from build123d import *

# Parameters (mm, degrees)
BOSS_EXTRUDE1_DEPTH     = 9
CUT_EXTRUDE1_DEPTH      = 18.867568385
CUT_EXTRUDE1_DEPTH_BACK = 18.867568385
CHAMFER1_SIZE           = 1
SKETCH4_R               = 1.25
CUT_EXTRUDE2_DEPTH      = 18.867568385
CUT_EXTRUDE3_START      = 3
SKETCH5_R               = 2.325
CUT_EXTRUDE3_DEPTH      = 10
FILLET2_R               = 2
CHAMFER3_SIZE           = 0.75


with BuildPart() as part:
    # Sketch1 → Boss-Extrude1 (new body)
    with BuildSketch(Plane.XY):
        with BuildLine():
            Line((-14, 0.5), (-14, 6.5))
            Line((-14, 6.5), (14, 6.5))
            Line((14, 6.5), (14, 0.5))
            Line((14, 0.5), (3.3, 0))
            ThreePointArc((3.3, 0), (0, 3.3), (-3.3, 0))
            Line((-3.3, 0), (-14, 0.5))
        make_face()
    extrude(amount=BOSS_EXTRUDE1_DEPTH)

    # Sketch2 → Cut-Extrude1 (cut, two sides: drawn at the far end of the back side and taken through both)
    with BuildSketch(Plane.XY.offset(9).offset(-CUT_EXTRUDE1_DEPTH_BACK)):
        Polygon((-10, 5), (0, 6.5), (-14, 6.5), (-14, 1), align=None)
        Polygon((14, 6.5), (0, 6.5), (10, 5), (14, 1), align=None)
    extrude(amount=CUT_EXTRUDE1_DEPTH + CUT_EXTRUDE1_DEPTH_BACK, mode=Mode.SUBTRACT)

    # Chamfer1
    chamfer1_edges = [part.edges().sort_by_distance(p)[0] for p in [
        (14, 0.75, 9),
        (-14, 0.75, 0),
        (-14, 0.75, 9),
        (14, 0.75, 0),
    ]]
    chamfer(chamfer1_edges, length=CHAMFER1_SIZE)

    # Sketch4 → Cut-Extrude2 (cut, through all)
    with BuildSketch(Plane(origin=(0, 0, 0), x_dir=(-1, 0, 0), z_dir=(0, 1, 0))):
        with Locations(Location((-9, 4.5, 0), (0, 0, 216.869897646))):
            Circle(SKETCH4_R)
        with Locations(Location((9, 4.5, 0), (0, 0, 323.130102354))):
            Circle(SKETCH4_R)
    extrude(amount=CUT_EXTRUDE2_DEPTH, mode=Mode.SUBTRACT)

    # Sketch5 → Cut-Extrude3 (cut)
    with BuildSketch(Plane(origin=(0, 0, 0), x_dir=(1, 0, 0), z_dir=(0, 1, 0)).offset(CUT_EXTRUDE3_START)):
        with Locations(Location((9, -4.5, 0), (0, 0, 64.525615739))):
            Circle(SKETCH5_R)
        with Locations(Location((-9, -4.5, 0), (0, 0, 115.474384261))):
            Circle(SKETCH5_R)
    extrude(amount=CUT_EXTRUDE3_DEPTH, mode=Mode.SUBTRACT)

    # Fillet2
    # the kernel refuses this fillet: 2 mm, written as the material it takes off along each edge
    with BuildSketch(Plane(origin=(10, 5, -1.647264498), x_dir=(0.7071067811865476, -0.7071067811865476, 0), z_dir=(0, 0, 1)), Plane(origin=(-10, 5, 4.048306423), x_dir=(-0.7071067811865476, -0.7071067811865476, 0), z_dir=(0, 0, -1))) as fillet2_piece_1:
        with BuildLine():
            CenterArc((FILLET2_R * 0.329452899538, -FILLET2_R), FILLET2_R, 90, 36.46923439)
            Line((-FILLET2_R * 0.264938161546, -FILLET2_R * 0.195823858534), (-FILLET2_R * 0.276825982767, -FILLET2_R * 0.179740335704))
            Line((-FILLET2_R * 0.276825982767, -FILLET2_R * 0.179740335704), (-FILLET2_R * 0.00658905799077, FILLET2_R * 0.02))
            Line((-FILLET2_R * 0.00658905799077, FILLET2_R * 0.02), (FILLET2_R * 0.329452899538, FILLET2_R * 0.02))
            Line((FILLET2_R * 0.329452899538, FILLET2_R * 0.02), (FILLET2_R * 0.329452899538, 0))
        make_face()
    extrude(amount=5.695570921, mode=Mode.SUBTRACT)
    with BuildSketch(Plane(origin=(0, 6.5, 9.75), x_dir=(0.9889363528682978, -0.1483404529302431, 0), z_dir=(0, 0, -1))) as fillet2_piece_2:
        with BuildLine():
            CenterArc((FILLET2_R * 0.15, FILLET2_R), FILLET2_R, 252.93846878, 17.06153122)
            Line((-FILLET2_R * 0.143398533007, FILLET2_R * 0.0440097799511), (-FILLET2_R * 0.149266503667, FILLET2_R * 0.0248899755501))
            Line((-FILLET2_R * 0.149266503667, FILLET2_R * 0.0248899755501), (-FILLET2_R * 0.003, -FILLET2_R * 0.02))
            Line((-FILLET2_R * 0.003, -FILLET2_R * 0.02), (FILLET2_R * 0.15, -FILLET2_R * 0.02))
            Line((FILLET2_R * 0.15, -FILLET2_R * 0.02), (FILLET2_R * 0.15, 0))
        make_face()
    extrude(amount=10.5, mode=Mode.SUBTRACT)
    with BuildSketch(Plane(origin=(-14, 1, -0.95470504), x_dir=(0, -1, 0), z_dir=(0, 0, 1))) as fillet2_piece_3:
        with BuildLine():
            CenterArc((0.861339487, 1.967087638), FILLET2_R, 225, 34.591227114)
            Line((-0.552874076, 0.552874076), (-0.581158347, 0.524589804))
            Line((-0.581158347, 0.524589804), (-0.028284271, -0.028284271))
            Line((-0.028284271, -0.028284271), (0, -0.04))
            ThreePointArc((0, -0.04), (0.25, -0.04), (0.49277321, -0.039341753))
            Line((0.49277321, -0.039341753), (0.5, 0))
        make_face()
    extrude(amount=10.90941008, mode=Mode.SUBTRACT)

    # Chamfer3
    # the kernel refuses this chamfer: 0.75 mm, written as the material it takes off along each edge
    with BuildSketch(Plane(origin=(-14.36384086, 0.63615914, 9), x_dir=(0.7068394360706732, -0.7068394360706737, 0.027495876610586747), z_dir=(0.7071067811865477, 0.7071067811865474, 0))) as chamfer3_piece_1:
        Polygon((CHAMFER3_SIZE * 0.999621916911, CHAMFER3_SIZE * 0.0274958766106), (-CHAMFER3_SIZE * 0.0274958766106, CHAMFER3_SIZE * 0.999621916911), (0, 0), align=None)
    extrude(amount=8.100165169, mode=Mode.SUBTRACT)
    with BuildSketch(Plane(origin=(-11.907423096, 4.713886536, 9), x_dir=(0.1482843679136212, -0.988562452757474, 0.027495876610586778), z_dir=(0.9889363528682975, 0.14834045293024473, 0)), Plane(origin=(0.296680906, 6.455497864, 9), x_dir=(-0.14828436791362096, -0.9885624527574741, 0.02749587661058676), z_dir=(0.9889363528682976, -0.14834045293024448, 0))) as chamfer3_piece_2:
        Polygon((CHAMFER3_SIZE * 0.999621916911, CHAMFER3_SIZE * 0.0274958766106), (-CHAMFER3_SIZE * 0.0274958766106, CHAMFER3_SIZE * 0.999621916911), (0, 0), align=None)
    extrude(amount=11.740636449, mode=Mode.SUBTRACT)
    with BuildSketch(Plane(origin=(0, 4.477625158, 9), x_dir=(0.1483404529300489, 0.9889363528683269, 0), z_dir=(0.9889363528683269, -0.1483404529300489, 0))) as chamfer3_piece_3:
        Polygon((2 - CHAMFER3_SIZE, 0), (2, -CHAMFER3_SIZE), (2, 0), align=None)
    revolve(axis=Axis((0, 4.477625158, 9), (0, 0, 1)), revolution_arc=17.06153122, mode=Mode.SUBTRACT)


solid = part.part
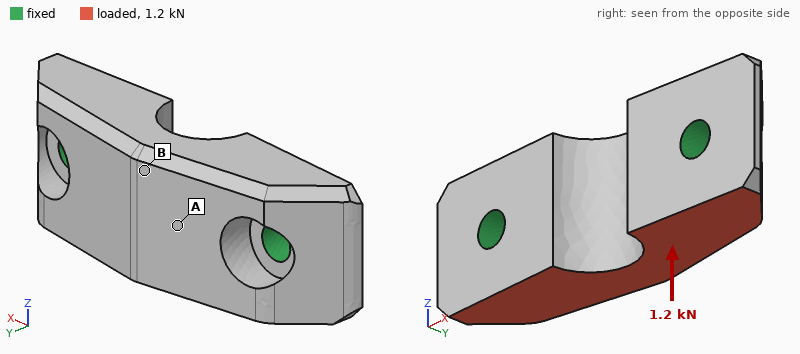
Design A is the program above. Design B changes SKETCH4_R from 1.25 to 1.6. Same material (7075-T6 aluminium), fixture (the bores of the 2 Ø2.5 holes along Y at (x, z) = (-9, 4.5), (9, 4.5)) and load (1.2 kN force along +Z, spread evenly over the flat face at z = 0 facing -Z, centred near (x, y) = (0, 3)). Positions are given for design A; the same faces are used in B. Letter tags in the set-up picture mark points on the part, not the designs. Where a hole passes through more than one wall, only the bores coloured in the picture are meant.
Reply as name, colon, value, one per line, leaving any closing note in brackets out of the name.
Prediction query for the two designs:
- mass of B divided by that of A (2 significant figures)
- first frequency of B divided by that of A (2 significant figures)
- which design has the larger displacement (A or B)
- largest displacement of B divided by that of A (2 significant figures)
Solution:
mass of B divided by that of A: 0.98
first frequency of B divided by that of A: 1.2
which design has the larger displacement: A
largest displacement of B divided by that of A: 0.78
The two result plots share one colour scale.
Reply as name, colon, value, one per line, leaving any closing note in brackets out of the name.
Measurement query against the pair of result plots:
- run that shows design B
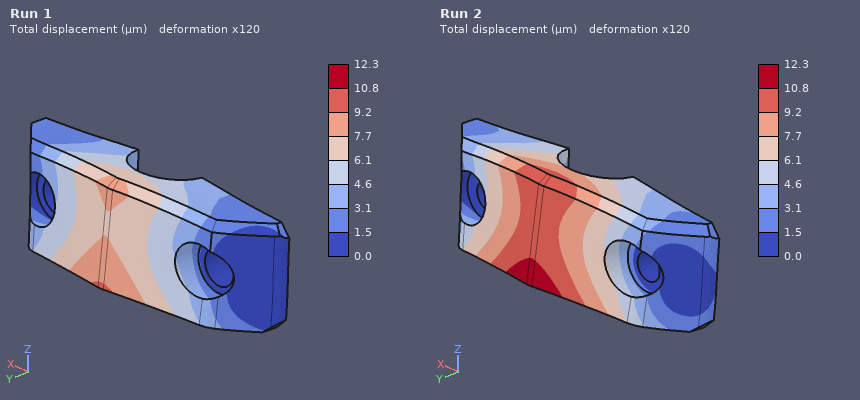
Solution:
run that shows design B: Run 1
